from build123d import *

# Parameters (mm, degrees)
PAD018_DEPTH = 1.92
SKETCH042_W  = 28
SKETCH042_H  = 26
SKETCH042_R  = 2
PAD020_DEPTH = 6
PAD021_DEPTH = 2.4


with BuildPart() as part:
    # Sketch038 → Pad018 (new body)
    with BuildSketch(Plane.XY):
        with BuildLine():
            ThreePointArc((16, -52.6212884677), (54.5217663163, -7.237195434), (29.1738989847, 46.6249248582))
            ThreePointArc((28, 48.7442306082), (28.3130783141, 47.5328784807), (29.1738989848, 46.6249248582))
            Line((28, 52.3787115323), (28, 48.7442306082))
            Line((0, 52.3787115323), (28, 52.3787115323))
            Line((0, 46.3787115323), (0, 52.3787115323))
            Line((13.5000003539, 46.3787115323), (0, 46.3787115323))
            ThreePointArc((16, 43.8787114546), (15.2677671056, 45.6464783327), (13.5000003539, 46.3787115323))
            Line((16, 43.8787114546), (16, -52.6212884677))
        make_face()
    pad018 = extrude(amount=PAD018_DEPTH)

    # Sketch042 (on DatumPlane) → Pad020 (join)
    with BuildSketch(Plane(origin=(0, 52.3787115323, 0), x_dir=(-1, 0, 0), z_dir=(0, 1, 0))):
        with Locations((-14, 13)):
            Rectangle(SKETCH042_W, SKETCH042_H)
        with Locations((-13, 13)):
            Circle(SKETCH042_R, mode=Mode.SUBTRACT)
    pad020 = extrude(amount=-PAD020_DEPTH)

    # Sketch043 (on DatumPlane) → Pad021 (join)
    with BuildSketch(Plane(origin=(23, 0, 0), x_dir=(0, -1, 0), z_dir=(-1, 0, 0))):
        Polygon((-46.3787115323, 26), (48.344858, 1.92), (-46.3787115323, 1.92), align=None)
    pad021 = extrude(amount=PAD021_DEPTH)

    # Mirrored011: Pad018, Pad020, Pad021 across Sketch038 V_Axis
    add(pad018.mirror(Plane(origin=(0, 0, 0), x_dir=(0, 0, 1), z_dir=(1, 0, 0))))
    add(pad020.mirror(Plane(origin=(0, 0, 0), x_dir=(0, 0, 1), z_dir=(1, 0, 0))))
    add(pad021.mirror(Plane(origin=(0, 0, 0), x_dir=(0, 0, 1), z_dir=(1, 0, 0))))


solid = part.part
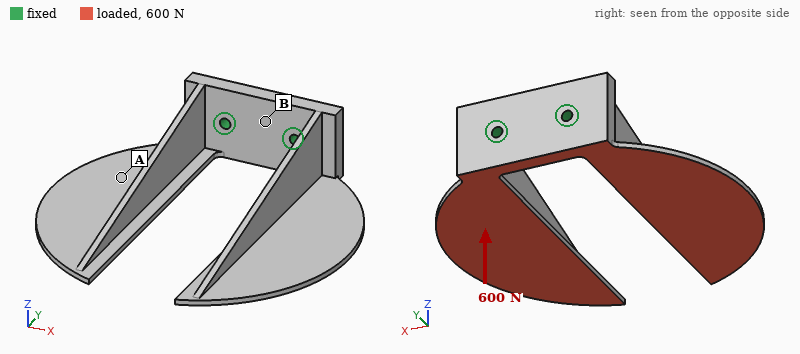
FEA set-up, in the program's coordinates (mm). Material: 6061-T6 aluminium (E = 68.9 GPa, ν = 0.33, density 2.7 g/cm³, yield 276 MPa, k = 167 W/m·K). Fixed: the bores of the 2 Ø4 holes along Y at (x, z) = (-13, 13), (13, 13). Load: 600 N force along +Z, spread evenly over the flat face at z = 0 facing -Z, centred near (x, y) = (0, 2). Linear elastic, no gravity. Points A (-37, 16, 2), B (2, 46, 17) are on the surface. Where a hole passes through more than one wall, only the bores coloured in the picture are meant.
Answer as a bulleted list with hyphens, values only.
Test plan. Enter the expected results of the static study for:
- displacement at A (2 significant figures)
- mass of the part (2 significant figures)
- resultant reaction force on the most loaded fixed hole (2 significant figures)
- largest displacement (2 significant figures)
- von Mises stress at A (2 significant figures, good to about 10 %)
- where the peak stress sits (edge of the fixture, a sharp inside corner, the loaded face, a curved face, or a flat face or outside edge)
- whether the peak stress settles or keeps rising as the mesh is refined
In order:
- 0.42 mm
- 69 g
- 300 N
- 1.3 mm
- 39 MPa
- edge of the fixture
- keeps rising
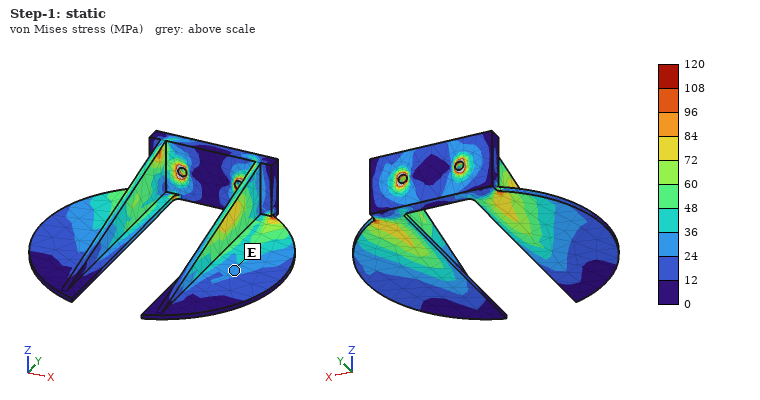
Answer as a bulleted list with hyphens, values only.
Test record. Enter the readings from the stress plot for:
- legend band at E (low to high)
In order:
- 24 to 36 MPa
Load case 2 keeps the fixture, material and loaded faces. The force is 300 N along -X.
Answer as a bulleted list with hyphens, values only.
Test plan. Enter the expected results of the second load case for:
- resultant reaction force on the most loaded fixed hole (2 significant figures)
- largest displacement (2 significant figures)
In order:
- 280 N
- 0.58 mm
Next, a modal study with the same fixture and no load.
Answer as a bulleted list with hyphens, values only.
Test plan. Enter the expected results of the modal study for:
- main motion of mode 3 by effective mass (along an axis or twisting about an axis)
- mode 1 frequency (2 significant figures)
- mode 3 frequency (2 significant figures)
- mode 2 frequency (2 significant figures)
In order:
- along Z
- 690 Hz
- 790 Hz
- 710 Hz
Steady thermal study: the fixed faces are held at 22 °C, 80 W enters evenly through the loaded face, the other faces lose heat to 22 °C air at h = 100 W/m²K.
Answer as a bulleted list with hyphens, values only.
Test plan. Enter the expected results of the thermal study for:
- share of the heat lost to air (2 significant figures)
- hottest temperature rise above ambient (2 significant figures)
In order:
- 58 %
- 57 K
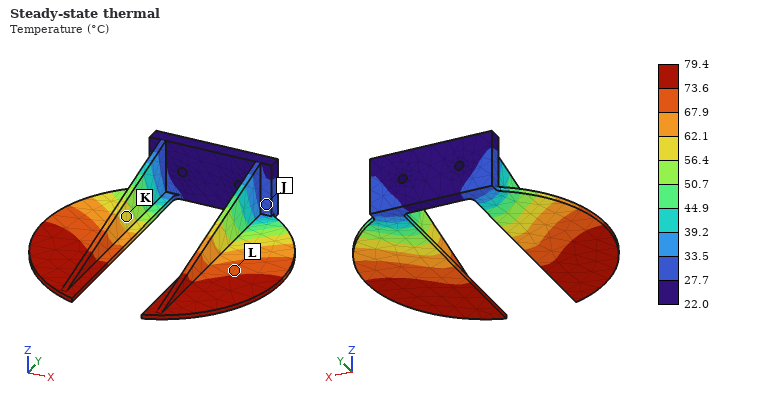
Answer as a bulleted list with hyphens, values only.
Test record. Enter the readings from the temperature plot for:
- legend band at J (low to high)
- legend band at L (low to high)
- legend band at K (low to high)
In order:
- 27.7 to 33.5 °C
- 67.9 to 73.6 °C
- 56.4 to 62.1 °C
